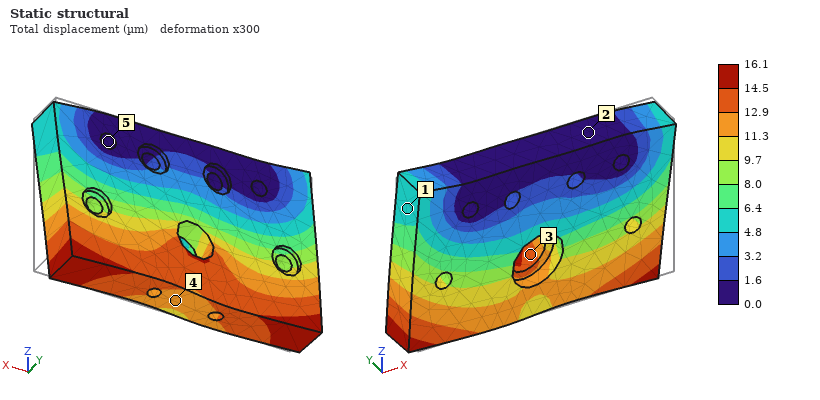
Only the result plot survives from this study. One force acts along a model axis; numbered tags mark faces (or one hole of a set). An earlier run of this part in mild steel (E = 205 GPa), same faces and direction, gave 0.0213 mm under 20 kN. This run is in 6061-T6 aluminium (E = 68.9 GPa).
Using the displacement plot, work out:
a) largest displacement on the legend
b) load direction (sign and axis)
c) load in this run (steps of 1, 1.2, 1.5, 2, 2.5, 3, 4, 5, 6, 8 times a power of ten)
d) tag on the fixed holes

16.1 µm
-X
5 kN
5
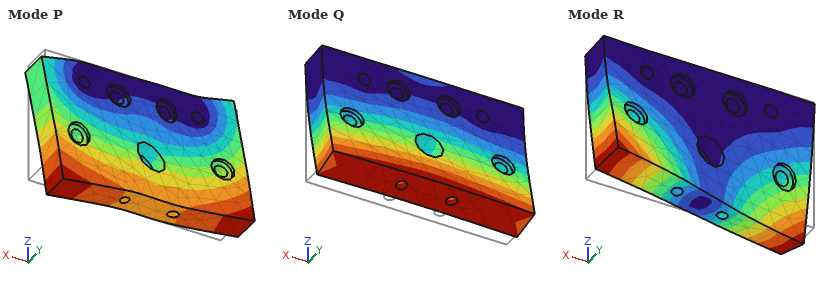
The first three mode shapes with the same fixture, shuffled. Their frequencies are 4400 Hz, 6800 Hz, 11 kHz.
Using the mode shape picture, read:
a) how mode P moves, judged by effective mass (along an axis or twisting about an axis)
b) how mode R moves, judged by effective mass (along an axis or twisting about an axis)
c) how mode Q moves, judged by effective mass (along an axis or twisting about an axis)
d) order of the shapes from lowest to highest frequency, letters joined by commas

along X
twisting about Z
along Y
Q, R, P
